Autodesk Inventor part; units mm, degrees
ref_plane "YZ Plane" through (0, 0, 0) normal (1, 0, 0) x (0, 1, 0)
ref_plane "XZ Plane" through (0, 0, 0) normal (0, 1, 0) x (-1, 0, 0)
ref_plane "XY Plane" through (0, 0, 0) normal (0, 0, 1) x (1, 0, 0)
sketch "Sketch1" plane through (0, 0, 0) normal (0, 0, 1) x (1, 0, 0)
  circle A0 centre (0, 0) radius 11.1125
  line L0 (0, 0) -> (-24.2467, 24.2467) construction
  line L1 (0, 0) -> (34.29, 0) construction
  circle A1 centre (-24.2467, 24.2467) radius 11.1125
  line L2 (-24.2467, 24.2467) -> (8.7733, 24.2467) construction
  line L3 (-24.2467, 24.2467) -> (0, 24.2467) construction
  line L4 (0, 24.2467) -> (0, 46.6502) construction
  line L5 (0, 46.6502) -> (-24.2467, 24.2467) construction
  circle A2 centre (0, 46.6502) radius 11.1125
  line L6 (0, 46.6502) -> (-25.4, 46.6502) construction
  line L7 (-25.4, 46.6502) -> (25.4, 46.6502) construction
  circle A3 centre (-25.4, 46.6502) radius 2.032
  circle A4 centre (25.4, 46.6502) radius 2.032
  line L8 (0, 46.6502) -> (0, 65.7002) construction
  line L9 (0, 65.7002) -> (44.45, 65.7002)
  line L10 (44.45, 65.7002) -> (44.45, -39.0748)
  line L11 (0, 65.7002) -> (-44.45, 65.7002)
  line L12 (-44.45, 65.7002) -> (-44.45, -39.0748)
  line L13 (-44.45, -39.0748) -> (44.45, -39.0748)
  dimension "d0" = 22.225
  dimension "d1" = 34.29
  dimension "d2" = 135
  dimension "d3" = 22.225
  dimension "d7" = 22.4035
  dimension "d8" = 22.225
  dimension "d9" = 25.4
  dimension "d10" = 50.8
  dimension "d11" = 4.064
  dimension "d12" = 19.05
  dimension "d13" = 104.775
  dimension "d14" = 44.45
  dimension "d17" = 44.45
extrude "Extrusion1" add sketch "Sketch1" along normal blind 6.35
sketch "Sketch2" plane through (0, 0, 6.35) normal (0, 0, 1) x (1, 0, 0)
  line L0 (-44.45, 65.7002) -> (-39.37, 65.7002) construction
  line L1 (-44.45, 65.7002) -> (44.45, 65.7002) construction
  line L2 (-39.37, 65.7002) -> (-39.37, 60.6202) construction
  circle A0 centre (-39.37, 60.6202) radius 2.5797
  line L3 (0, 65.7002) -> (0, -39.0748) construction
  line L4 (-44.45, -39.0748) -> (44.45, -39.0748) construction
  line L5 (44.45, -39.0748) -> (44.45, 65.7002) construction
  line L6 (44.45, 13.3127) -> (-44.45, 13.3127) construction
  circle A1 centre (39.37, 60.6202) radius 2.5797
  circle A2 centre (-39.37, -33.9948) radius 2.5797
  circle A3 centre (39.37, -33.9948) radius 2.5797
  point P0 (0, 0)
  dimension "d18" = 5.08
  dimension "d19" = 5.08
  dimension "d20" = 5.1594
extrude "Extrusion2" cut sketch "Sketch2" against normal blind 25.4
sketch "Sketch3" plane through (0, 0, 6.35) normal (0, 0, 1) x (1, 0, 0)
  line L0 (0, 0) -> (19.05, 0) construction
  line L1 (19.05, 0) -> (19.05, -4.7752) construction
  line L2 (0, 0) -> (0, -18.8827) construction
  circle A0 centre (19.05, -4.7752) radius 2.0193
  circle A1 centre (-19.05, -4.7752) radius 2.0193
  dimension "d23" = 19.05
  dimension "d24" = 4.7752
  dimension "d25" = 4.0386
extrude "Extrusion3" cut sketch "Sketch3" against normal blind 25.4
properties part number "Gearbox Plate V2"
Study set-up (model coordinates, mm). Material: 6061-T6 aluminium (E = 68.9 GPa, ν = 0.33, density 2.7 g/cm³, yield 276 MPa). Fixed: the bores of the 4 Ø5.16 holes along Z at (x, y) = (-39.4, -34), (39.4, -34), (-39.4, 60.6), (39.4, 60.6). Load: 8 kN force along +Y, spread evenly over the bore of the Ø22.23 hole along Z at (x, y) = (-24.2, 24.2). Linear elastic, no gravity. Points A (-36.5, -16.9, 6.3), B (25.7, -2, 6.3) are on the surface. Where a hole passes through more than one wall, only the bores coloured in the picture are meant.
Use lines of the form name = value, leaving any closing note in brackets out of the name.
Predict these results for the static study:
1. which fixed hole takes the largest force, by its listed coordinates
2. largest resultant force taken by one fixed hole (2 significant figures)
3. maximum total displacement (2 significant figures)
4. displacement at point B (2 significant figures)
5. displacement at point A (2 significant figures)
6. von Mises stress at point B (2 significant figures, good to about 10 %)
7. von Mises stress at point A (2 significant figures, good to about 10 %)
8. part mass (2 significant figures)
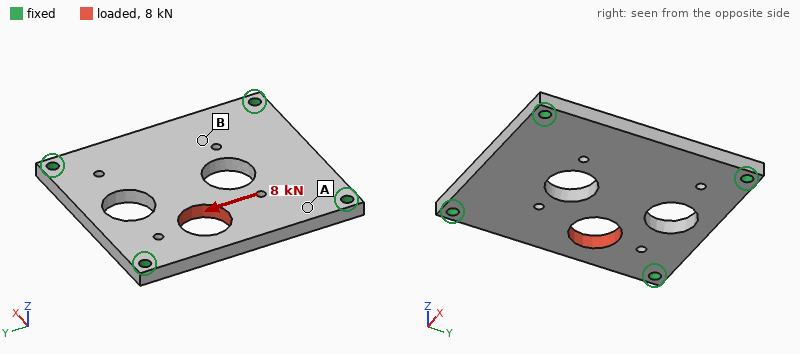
which fixed hole takes the largest force, by its listed coordinates = (-39.4, 60.6)
largest resultant force taken by one fixed hole = 3.5 kN
maximum total displacement = 23 µm
displacement at point B = 3.8 µm
displacement at point A = 7.0 µm
von Mises stress at point B = 7.2 MPa
von Mises stress at point A = 21 MPa
part mass = 140 g
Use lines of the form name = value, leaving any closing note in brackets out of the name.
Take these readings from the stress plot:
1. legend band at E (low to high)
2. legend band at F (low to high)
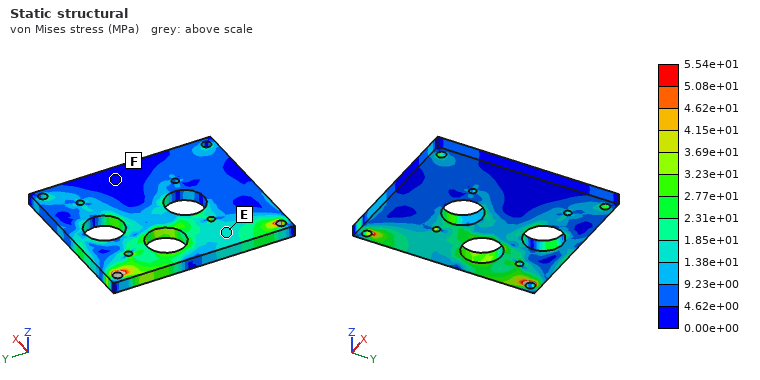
legend band at E = 1.38e+01 to 1.85e+01 MPa
legend band at F = 0.00e+00 to 4.62e+00 MPa
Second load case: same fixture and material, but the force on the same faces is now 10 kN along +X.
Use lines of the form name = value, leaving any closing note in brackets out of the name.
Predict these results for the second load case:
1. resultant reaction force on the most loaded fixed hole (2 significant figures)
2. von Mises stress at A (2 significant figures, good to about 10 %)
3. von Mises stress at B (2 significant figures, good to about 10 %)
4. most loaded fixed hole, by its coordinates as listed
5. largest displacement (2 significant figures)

resultant reaction force on the most loaded fixed hole = 3.6 kN
von Mises stress at A = 13 MPa
von Mises stress at B = 16 MPa
most loaded fixed hole, by its coordinates as listed = (-39.4, 60.6)
largest displacement = 57 µm
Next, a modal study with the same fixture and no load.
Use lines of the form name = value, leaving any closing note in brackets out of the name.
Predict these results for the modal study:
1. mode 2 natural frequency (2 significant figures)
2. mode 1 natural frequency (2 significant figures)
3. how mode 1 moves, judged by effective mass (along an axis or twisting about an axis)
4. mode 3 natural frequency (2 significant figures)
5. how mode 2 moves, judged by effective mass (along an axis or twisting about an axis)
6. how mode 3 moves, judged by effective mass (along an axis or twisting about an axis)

mode 2 natural frequency = 4200 Hz
mode 1 natural frequency = 2600 Hz
how mode 1 moves, judged by effective mass = along Z
mode 3 natural frequency = 5100 Hz
how mode 2 moves, judged by effective mass = twisting about Y
how mode 3 moves, judged by effective mass = twisting about X
